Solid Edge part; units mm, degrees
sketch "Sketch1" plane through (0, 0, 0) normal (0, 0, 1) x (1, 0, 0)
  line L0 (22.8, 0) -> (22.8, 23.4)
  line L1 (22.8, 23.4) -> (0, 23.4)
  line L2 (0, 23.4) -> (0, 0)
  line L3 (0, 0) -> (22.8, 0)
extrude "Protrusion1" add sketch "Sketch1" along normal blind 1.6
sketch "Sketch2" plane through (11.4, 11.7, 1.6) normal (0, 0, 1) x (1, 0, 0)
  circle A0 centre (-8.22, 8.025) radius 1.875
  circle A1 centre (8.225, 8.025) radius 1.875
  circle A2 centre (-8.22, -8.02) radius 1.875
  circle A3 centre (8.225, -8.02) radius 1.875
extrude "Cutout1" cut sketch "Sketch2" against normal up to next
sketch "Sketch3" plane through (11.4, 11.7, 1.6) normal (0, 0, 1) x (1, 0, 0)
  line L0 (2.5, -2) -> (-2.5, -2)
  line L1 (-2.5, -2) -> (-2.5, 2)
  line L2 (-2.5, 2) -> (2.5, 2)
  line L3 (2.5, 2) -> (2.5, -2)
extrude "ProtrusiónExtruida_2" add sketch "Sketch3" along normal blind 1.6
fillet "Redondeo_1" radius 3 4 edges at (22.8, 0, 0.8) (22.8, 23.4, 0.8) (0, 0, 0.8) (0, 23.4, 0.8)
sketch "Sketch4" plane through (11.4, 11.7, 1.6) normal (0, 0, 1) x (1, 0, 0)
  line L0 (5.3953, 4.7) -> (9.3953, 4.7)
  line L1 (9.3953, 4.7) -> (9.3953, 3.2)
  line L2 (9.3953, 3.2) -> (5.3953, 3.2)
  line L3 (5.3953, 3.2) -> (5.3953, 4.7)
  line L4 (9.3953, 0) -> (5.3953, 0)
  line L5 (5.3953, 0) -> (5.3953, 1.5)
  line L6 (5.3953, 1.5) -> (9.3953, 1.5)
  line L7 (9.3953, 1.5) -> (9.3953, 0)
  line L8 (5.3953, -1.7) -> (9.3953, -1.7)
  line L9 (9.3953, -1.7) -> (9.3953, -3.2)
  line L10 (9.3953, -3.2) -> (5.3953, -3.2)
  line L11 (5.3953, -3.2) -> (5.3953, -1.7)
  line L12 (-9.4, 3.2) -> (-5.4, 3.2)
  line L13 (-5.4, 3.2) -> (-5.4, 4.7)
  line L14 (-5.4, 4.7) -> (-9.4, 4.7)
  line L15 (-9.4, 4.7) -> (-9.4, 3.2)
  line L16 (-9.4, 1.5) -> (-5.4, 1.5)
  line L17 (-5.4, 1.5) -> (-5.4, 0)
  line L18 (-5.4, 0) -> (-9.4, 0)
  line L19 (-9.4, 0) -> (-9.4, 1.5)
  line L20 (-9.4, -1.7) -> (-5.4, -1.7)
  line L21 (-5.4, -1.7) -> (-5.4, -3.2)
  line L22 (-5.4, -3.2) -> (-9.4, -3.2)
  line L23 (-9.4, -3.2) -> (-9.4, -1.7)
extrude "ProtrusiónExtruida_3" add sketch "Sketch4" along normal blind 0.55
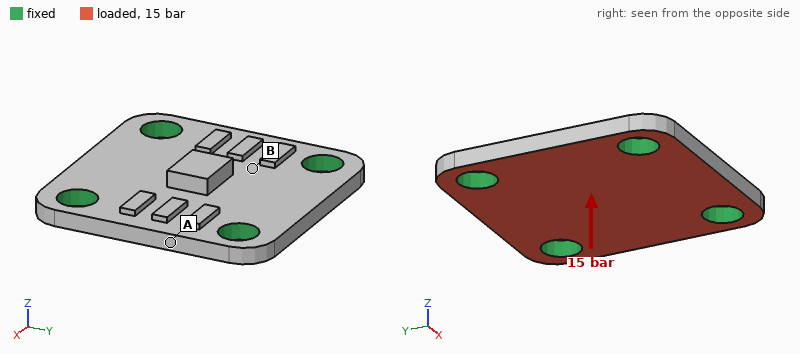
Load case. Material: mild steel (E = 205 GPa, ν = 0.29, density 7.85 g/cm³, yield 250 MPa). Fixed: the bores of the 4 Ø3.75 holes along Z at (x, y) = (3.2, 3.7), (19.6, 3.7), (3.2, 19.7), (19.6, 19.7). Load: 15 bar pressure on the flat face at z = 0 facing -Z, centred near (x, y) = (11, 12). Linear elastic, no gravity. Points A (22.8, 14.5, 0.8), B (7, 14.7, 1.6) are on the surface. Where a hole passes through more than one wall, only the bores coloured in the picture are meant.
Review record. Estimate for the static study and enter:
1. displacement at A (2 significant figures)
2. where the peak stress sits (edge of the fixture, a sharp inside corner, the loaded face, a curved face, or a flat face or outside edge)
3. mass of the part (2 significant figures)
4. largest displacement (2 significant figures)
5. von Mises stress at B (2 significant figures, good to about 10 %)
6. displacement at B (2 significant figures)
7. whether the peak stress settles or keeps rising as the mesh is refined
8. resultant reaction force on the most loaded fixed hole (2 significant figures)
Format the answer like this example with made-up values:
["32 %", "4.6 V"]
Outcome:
["1.1 µm", "edge of the fixture", "6.5 g", "4.3 µm", "19 MPa", "3.1 µm", "keeps rising", "180 N"]
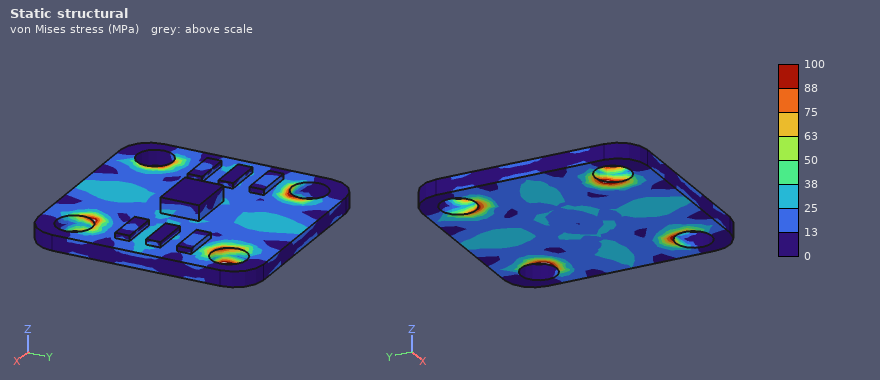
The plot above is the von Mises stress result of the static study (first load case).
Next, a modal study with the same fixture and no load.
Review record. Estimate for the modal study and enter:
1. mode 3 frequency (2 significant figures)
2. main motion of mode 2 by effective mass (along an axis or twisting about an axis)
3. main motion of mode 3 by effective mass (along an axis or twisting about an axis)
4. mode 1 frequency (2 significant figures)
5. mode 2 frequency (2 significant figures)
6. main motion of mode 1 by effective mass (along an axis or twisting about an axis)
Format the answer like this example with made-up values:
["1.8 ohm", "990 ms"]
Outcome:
["45 kHz", "twisting about X", "twisting about Y", "29 kHz", "43 kHz", "along Z"]
